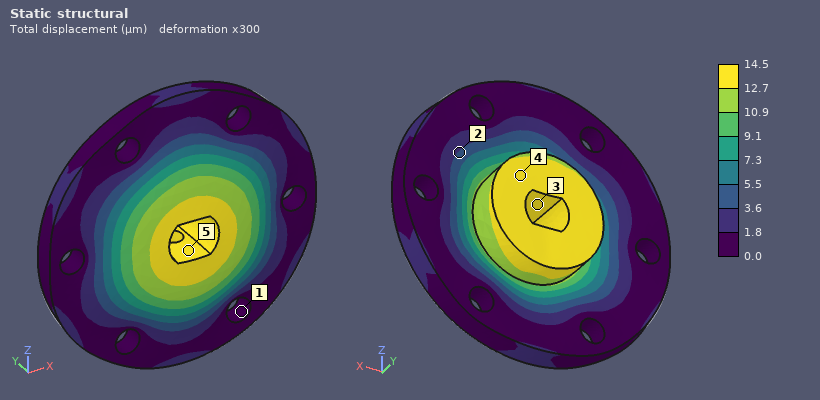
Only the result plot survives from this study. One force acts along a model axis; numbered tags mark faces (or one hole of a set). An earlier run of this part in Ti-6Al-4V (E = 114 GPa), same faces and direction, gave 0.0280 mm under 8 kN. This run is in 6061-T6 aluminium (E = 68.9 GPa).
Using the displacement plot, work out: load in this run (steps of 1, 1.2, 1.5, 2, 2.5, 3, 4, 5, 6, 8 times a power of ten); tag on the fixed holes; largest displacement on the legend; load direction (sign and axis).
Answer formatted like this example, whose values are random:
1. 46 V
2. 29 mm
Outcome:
1. 2.5 kN
2. 1
3. 14.5 µm
4. -Y
